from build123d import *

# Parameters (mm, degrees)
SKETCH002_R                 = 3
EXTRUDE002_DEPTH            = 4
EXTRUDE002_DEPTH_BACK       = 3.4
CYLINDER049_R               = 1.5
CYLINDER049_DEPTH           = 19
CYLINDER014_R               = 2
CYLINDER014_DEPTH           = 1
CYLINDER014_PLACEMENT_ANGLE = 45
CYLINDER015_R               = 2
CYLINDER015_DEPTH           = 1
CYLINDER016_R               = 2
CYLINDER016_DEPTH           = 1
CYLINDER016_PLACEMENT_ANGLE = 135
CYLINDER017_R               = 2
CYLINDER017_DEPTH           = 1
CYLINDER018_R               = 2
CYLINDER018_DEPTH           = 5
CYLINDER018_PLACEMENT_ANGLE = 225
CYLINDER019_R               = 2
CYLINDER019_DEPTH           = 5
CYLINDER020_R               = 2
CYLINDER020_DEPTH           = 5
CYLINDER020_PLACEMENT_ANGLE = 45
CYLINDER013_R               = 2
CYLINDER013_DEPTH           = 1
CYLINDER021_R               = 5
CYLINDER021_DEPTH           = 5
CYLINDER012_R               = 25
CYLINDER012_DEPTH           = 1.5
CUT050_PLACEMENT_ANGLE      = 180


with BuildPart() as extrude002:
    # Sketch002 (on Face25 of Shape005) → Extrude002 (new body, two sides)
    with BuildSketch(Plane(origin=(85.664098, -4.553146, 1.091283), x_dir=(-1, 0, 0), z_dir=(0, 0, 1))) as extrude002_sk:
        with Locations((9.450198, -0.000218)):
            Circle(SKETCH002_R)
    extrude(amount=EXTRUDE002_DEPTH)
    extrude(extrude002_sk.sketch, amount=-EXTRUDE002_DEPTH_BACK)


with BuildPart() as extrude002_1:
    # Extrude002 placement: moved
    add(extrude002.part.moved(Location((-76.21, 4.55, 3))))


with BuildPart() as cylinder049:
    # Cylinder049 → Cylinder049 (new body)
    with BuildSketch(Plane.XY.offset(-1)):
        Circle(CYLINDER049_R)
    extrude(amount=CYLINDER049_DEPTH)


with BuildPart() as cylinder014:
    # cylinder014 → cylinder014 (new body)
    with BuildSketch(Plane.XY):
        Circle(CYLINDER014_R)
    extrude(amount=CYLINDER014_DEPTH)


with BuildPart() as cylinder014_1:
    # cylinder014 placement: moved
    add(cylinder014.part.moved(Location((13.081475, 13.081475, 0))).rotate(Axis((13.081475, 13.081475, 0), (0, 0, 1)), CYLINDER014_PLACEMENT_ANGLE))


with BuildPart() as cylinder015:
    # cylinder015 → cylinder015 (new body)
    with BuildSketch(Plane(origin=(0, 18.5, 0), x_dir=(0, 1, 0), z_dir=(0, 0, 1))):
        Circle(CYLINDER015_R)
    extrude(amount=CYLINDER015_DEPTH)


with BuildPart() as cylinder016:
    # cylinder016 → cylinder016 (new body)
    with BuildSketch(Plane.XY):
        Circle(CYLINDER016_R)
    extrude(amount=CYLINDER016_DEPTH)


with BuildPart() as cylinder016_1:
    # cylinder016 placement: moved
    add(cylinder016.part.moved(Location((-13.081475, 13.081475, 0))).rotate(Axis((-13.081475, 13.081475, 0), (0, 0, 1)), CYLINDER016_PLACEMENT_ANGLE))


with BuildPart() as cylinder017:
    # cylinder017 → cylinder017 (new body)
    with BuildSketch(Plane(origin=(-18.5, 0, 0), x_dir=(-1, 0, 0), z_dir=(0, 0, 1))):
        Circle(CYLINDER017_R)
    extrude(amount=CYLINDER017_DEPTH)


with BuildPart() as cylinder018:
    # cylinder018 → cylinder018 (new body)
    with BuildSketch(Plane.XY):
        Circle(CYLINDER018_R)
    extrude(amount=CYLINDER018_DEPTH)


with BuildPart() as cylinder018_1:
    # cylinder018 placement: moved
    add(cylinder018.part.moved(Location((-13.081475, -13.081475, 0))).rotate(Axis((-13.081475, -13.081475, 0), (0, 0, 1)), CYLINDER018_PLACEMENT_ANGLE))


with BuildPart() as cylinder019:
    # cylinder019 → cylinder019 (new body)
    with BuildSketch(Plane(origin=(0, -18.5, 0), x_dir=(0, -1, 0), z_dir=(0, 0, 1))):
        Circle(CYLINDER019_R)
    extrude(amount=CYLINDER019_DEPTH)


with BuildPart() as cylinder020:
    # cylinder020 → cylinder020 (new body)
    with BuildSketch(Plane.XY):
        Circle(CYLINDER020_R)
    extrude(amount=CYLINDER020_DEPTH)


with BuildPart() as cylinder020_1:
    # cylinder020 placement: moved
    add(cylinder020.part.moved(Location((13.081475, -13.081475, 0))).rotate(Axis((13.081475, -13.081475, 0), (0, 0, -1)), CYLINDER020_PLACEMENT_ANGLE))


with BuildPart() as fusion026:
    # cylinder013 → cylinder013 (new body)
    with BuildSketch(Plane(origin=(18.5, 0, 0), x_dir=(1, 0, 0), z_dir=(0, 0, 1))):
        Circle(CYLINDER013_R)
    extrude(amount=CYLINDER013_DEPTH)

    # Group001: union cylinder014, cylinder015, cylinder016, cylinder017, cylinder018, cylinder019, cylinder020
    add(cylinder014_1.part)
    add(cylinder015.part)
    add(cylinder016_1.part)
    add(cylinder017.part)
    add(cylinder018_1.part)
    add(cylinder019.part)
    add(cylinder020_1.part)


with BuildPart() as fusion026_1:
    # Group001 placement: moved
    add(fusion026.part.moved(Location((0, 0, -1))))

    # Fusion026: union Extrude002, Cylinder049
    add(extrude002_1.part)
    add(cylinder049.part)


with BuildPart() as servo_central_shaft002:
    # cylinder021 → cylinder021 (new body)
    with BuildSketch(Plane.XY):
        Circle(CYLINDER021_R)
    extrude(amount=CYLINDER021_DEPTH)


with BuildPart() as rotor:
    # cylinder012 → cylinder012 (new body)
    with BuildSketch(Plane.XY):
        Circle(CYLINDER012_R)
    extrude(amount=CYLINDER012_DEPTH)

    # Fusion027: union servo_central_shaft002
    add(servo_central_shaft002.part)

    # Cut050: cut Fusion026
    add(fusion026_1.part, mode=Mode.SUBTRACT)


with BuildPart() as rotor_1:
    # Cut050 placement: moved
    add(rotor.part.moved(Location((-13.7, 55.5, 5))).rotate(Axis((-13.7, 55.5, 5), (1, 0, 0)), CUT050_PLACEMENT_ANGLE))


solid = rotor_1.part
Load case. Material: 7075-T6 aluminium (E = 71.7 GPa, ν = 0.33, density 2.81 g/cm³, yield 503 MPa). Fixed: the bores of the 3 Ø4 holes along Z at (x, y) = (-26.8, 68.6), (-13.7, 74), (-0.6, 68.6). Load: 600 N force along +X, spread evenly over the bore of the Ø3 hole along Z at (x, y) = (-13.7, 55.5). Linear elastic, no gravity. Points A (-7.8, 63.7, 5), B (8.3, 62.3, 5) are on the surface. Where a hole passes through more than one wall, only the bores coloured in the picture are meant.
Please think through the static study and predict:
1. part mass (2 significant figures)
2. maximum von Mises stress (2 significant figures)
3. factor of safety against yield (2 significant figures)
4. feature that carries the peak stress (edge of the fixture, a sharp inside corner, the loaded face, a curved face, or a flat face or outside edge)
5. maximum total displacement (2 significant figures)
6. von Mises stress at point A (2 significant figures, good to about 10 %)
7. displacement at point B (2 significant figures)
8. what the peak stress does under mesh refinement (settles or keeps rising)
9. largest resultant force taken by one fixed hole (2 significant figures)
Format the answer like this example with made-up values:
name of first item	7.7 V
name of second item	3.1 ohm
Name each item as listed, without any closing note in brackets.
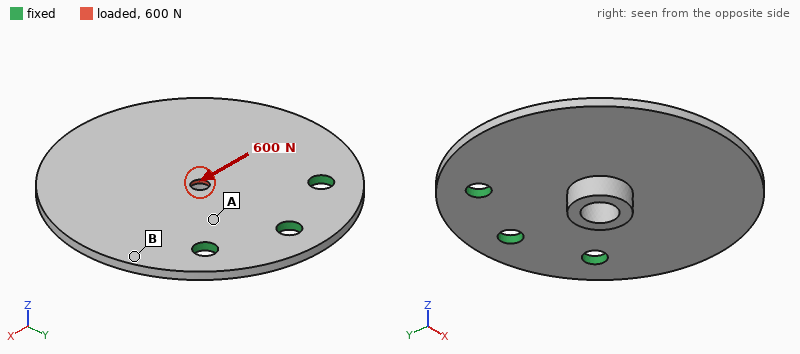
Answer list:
part mass	8.5 g
maximum von Mises stress	160 MPa
factor of safety against yield	3.1
feature that carries the peak stress	the loaded face
maximum total displacement	20 µm
von Mises stress at point A	26 MPa
displacement at point B	5.6 µm
what the peak stress does under mesh refinement	settles
largest resultant force taken by one fixed hole	380 N
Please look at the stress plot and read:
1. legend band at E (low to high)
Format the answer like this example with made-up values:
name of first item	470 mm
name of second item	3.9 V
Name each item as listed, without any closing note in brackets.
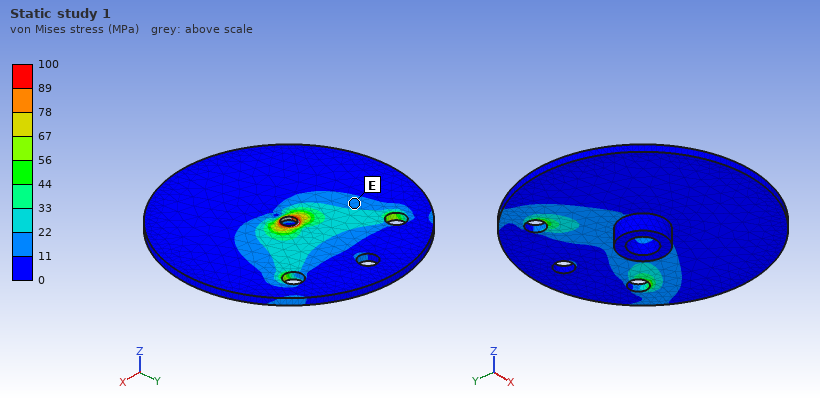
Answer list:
legend band at E	11 to 22 MPa
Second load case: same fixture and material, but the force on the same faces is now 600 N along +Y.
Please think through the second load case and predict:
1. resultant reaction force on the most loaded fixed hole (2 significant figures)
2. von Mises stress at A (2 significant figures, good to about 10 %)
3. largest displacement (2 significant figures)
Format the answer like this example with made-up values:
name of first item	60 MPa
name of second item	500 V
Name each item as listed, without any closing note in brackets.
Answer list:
resultant reaction force on the most loaded fixed hole	220 N
von Mises stress at A	24 MPa
largest displacement	92 µm
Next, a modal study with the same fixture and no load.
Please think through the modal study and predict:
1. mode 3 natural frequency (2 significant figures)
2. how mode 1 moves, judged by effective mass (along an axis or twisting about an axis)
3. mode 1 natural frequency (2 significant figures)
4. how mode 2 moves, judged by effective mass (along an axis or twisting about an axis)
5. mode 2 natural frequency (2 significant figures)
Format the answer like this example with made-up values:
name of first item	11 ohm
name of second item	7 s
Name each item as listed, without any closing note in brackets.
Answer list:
mode 3 natural frequency	4900 Hz
how mode 1 moves, judged by effective mass	along Z
mode 1 natural frequency	1100 Hz
how mode 2 moves, judged by effective mass	twisting about Y
mode 2 natural frequency	2600 Hz
